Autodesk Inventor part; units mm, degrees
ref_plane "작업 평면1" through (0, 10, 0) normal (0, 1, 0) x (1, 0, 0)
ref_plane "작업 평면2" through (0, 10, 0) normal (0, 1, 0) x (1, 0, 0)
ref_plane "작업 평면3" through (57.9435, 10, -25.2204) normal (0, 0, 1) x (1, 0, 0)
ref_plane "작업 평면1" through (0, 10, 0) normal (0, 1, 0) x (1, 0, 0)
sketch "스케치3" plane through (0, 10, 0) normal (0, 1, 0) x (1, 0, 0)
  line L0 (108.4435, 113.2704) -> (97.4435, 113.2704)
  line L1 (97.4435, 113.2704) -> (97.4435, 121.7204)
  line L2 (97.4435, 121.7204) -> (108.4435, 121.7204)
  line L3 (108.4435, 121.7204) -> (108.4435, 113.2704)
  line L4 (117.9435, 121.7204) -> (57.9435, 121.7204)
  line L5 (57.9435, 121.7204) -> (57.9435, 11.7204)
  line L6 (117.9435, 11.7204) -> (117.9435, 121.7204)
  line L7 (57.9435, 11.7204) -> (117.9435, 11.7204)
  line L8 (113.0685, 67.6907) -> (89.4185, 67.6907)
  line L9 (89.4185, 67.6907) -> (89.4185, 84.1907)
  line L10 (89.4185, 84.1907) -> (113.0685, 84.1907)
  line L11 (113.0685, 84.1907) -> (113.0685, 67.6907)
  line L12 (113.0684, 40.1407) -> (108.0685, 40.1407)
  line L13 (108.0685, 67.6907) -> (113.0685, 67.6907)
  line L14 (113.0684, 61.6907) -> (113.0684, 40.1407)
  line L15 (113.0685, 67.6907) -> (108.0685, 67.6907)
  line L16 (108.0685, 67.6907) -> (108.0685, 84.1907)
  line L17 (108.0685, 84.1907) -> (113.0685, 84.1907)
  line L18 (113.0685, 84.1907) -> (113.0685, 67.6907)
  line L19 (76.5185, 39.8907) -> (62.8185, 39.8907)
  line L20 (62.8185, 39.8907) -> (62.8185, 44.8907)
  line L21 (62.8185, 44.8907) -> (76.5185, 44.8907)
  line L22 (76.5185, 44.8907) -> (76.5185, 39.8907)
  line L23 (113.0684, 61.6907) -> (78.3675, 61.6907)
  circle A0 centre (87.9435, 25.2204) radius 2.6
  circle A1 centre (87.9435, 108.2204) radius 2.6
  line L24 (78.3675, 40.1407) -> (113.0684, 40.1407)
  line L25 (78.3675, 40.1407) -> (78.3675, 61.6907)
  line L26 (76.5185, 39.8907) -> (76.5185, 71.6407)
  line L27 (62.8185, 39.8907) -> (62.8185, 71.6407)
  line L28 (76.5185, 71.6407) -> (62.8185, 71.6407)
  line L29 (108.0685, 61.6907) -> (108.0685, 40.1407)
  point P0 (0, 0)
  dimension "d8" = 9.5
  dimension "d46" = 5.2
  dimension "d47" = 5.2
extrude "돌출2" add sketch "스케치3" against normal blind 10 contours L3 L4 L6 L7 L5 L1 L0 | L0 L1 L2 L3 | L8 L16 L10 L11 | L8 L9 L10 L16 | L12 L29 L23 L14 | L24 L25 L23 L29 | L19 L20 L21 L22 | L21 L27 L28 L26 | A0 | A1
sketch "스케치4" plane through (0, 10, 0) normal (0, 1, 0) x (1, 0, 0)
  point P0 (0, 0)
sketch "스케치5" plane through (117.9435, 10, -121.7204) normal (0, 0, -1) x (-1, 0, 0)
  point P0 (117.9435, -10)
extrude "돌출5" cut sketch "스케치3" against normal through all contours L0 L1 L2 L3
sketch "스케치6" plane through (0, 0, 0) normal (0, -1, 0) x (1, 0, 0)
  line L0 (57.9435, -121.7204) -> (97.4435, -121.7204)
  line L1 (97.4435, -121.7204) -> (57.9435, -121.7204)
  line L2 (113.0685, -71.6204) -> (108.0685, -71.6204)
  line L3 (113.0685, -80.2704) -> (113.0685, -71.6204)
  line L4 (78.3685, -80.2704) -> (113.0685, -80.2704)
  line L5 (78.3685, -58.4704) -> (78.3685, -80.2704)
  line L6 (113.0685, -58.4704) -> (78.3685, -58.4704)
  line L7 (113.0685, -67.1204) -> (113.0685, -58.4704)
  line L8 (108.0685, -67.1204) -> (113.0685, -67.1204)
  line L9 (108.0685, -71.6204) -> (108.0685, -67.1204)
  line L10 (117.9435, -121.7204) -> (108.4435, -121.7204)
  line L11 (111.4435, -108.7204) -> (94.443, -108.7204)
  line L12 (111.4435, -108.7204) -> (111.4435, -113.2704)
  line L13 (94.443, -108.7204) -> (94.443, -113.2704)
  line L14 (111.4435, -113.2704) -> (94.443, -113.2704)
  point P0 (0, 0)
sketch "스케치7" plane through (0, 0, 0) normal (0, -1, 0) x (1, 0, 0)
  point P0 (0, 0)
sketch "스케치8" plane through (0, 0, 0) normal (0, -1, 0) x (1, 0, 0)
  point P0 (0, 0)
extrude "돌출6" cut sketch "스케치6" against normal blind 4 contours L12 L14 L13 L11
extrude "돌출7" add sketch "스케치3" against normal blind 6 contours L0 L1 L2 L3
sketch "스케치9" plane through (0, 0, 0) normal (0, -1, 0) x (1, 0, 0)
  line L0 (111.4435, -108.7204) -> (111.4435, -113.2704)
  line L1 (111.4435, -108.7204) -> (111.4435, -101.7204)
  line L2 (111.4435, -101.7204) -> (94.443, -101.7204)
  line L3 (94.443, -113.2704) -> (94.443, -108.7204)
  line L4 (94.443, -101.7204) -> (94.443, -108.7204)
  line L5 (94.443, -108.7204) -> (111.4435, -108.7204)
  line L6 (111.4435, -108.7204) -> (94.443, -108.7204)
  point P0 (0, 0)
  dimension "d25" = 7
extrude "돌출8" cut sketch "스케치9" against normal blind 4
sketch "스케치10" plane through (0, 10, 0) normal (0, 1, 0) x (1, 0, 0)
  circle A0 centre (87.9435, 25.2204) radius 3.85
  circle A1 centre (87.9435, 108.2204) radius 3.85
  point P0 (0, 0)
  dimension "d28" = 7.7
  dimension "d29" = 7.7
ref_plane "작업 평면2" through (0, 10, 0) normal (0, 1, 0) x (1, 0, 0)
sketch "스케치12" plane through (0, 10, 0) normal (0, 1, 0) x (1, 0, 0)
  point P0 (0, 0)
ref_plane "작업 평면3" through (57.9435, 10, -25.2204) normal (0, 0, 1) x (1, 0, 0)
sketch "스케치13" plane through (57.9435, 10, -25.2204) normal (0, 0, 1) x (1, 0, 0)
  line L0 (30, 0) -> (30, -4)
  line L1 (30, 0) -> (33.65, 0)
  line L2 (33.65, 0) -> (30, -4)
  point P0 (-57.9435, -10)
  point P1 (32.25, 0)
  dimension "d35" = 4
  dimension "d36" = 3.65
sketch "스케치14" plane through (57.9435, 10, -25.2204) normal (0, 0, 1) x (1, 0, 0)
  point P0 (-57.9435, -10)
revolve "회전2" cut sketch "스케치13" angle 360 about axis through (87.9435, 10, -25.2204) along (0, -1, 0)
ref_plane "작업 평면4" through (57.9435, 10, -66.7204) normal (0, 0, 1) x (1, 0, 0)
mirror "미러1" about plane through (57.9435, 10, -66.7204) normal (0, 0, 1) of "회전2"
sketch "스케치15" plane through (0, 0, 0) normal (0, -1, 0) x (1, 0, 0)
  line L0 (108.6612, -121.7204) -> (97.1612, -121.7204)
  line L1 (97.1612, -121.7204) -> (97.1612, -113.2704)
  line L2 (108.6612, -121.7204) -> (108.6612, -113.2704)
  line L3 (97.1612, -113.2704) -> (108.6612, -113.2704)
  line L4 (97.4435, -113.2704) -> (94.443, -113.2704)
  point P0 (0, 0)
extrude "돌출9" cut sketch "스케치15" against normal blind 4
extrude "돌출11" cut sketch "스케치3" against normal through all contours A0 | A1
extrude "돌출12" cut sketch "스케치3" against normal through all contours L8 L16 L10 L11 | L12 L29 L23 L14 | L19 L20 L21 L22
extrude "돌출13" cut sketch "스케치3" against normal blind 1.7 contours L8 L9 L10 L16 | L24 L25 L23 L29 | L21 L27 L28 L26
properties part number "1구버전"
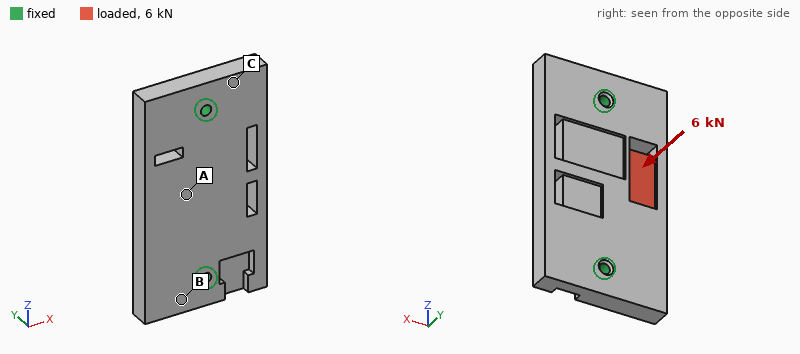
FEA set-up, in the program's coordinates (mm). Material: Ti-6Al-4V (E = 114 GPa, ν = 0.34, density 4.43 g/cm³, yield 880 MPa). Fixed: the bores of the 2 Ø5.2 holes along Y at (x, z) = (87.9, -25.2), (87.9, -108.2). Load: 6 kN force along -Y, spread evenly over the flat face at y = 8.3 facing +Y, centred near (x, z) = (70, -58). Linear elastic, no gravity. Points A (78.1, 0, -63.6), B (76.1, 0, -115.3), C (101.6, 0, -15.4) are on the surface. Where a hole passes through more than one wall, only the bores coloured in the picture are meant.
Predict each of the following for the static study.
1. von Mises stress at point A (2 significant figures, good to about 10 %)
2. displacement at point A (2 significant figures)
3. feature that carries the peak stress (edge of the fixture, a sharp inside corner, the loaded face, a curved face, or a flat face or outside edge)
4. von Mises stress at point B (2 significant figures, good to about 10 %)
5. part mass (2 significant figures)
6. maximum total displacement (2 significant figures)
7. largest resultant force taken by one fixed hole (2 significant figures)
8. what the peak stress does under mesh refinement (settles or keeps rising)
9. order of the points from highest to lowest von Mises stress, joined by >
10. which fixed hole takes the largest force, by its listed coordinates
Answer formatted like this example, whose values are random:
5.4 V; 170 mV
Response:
77 MPa; 0.095 mm; edge of the fixture; 51 MPa; 260 g; 0.17 mm; 3.8 kN; keeps rising; A > B > C; (87.9, -25.2)
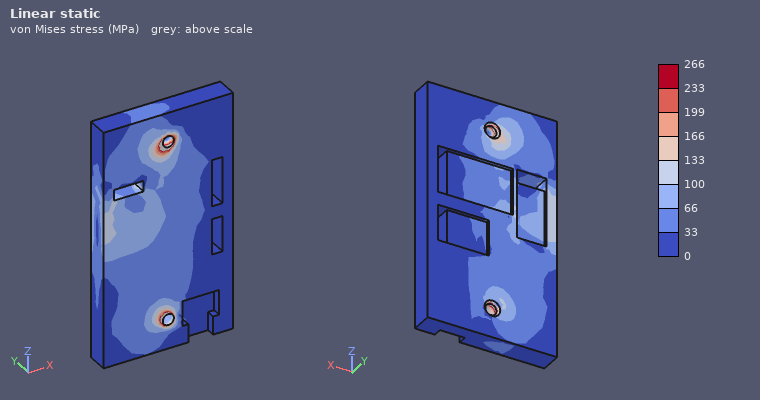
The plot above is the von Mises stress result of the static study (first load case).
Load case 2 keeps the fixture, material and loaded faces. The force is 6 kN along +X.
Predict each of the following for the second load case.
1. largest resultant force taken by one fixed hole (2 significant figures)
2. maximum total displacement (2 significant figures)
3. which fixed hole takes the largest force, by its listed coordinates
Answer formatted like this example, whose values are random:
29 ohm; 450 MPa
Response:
3.6 kN; 36 µm; (87.9, -25.2)
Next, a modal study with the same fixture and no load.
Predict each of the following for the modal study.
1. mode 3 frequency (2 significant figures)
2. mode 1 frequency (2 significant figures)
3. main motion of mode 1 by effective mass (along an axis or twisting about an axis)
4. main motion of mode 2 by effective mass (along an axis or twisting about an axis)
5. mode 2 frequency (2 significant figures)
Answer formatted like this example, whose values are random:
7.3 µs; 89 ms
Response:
7000 Hz; 4200 Hz; twisting about Z; along Y; 4800 Hz
